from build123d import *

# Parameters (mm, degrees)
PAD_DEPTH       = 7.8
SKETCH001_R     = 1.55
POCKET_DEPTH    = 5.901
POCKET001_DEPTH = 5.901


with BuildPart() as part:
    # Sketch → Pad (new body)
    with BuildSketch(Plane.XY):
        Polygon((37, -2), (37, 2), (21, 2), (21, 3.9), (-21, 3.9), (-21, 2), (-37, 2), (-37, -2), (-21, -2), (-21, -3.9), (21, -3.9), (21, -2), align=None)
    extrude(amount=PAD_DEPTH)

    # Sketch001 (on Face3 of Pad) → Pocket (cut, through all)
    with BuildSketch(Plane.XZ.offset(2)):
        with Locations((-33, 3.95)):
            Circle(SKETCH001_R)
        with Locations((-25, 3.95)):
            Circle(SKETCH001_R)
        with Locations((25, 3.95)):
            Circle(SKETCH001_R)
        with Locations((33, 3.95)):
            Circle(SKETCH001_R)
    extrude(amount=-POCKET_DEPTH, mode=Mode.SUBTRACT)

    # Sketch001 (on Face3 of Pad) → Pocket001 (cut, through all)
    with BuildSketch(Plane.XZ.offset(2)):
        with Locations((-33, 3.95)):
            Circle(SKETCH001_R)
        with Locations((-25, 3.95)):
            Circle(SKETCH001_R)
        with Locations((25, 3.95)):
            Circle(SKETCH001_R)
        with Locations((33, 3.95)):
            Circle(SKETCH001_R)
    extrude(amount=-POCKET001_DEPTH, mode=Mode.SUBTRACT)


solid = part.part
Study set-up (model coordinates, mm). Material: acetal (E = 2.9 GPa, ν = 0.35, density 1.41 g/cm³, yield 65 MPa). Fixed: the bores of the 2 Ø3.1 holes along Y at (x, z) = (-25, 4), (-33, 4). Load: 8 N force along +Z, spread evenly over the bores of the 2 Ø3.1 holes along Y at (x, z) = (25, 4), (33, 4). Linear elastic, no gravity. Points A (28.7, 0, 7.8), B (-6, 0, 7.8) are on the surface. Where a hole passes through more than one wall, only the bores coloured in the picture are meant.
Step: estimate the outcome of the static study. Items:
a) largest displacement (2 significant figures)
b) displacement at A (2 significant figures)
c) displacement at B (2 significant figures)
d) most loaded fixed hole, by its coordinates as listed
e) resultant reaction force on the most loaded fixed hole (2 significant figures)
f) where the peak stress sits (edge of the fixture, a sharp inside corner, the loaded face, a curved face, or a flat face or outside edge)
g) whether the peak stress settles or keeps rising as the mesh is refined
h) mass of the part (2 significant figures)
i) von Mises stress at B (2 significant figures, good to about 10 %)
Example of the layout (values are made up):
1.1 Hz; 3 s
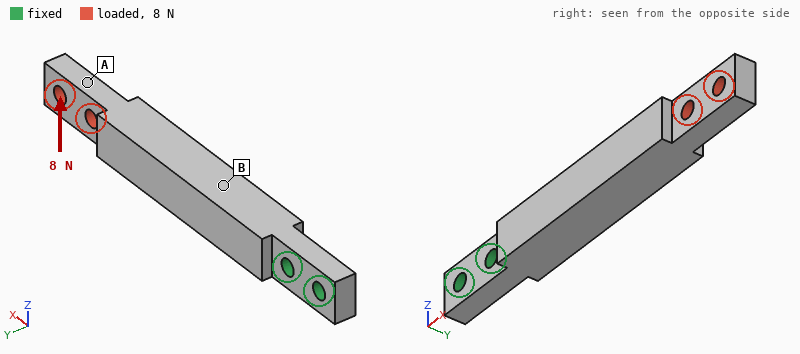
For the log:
0.82 mm; 0.67 mm; 0.15 mm; (-25, 4); 26 N; edge of the fixture; keeps rising; 4.8 g; 3.5 MPa
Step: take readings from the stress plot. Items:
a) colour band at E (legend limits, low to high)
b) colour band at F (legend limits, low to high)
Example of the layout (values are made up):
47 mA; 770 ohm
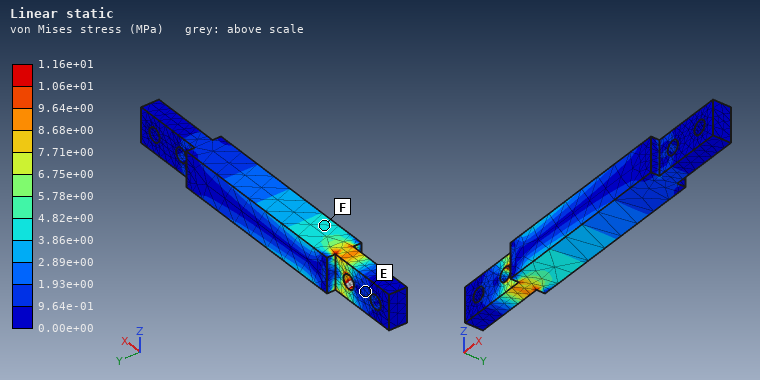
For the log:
9.64e-01 to 1.93e+00 MPa; 3.86e+00 to 4.82e+00 MPa
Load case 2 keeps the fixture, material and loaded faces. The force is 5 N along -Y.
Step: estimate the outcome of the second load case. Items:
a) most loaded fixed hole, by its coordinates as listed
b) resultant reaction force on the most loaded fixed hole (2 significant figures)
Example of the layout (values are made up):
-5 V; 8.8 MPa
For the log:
(-25, 4); 8.8 N
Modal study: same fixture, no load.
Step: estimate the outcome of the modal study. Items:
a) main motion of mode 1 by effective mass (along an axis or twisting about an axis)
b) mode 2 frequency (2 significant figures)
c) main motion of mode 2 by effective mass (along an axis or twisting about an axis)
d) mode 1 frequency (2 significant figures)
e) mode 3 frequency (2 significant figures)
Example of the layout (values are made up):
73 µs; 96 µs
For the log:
along Y; 480 Hz; along Z; 370 Hz; 2300 Hz
